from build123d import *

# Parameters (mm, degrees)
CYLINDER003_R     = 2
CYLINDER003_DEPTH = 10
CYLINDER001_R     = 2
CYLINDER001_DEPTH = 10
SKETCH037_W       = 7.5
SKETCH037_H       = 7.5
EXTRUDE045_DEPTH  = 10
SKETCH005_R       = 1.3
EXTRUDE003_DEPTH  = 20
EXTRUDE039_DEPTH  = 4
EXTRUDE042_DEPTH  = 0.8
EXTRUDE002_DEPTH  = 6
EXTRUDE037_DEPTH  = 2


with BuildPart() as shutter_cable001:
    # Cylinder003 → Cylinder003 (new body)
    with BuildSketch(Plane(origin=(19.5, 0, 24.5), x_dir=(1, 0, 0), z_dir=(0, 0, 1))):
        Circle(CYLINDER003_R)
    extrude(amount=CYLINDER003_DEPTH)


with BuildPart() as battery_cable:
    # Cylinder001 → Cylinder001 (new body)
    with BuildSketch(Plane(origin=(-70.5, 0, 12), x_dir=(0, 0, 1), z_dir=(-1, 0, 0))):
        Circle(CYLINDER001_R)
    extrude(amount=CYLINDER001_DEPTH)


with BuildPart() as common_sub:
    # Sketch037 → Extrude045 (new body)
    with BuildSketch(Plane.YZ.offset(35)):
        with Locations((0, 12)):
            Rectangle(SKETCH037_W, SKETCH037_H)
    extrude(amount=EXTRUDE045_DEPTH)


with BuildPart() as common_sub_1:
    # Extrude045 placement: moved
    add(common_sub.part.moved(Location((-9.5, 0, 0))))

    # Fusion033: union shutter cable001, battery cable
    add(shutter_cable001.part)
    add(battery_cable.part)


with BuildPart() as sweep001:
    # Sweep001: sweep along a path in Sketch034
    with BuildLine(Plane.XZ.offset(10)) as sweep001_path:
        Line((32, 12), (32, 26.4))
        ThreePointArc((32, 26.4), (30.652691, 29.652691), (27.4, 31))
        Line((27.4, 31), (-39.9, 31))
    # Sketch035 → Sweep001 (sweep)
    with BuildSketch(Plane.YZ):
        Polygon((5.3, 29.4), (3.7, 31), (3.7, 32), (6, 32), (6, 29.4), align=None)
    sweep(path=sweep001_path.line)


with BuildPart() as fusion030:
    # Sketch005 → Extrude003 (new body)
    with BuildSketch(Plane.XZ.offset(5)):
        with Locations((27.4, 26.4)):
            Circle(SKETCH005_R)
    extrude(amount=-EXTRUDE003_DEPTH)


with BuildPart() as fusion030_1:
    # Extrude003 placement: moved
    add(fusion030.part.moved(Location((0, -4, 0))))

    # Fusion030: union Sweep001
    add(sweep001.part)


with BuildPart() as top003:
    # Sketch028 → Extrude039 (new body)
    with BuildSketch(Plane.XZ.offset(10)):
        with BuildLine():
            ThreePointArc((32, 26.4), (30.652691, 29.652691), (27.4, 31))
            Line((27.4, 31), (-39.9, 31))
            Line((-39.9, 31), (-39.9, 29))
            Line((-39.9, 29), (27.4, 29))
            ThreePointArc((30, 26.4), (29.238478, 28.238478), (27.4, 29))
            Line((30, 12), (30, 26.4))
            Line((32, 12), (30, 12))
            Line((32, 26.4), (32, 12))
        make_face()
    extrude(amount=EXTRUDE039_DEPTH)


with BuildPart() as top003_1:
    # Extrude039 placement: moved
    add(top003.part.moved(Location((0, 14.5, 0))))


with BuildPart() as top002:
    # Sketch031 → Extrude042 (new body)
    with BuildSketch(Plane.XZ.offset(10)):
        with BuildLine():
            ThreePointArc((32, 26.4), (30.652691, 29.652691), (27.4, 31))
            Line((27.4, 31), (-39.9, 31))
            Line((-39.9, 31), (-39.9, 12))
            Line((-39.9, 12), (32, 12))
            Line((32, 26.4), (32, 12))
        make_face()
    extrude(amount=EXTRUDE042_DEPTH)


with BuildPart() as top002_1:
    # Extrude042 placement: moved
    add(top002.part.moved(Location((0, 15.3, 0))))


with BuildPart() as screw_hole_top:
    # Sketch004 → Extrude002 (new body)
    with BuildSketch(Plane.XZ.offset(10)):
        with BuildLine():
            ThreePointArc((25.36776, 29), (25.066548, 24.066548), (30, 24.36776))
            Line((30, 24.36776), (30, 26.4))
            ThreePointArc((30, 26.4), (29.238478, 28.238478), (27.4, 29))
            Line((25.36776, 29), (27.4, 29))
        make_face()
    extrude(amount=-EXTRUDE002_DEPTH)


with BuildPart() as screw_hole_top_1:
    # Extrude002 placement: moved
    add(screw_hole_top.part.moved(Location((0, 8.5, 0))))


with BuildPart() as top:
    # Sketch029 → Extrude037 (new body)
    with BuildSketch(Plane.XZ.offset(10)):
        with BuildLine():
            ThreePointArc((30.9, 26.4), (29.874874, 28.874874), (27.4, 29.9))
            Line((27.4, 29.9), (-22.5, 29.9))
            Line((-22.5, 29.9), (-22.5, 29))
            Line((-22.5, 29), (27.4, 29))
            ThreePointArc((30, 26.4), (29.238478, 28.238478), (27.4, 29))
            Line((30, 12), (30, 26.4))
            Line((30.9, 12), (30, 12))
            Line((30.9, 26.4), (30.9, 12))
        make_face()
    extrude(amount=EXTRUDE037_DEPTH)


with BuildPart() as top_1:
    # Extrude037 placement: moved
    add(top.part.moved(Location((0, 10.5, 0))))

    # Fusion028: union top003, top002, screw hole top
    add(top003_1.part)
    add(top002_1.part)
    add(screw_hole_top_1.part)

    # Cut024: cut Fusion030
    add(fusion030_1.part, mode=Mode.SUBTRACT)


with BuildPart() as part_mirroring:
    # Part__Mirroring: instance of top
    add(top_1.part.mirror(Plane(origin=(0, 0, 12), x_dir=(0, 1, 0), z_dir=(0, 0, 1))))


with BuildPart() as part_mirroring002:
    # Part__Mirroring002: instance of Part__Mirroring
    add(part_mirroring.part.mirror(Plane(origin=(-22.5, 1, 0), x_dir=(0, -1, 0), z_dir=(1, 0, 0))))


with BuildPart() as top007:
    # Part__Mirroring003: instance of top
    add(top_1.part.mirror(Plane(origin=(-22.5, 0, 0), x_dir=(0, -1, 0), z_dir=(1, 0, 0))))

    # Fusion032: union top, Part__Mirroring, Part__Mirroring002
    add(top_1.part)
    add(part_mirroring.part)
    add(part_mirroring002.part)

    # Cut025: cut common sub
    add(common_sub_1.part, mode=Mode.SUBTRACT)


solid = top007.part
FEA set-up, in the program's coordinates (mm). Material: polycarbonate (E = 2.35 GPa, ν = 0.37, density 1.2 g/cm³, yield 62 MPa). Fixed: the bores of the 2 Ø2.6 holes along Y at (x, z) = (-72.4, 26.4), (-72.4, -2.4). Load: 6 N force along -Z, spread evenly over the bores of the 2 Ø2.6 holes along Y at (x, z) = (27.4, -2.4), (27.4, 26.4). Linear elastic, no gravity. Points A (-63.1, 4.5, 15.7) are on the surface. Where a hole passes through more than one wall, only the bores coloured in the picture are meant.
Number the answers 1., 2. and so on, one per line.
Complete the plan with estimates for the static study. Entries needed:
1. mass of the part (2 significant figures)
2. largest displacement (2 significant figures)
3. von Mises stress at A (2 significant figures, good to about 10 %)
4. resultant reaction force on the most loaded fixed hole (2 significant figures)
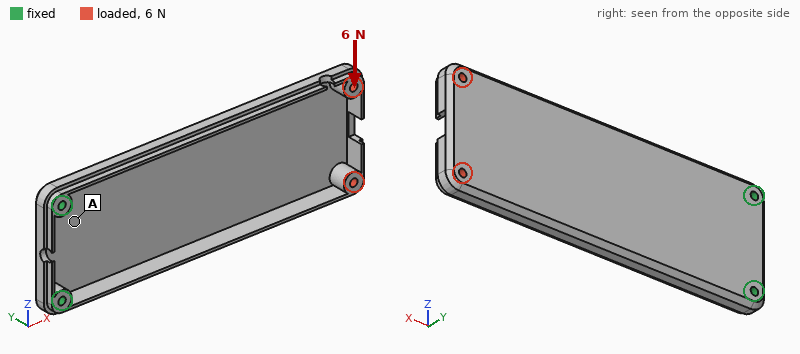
1. 7.4 g
2. 1.2 mm
3. 0.57 MPa
4. 20 N
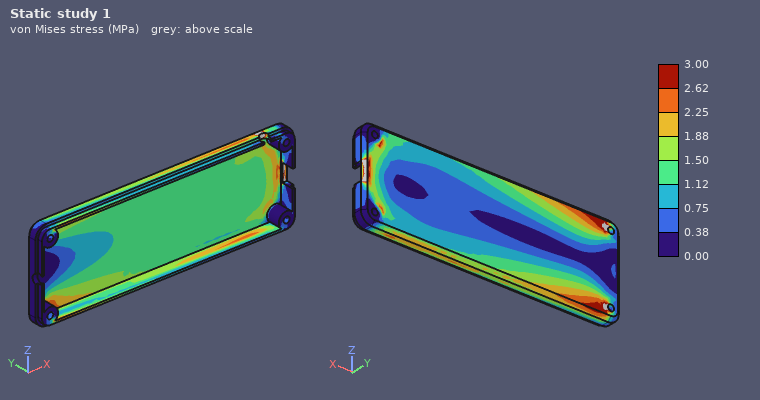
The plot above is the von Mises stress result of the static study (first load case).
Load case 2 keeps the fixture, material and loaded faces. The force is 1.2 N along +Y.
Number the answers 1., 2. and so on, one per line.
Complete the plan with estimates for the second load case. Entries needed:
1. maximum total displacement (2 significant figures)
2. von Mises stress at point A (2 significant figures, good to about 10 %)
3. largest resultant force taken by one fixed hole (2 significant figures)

1. 1.4 mm
2. 0.35 MPa
3. 2.1 N
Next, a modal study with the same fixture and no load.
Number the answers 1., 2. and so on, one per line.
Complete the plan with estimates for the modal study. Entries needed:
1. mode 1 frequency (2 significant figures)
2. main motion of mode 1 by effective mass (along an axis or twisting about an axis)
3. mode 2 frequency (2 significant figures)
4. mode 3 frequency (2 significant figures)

1. 100 Hz
2. along Y
3. 170 Hz
4. 520 Hz
